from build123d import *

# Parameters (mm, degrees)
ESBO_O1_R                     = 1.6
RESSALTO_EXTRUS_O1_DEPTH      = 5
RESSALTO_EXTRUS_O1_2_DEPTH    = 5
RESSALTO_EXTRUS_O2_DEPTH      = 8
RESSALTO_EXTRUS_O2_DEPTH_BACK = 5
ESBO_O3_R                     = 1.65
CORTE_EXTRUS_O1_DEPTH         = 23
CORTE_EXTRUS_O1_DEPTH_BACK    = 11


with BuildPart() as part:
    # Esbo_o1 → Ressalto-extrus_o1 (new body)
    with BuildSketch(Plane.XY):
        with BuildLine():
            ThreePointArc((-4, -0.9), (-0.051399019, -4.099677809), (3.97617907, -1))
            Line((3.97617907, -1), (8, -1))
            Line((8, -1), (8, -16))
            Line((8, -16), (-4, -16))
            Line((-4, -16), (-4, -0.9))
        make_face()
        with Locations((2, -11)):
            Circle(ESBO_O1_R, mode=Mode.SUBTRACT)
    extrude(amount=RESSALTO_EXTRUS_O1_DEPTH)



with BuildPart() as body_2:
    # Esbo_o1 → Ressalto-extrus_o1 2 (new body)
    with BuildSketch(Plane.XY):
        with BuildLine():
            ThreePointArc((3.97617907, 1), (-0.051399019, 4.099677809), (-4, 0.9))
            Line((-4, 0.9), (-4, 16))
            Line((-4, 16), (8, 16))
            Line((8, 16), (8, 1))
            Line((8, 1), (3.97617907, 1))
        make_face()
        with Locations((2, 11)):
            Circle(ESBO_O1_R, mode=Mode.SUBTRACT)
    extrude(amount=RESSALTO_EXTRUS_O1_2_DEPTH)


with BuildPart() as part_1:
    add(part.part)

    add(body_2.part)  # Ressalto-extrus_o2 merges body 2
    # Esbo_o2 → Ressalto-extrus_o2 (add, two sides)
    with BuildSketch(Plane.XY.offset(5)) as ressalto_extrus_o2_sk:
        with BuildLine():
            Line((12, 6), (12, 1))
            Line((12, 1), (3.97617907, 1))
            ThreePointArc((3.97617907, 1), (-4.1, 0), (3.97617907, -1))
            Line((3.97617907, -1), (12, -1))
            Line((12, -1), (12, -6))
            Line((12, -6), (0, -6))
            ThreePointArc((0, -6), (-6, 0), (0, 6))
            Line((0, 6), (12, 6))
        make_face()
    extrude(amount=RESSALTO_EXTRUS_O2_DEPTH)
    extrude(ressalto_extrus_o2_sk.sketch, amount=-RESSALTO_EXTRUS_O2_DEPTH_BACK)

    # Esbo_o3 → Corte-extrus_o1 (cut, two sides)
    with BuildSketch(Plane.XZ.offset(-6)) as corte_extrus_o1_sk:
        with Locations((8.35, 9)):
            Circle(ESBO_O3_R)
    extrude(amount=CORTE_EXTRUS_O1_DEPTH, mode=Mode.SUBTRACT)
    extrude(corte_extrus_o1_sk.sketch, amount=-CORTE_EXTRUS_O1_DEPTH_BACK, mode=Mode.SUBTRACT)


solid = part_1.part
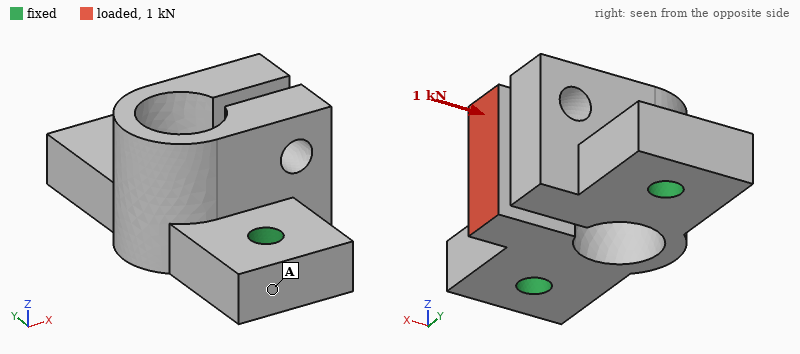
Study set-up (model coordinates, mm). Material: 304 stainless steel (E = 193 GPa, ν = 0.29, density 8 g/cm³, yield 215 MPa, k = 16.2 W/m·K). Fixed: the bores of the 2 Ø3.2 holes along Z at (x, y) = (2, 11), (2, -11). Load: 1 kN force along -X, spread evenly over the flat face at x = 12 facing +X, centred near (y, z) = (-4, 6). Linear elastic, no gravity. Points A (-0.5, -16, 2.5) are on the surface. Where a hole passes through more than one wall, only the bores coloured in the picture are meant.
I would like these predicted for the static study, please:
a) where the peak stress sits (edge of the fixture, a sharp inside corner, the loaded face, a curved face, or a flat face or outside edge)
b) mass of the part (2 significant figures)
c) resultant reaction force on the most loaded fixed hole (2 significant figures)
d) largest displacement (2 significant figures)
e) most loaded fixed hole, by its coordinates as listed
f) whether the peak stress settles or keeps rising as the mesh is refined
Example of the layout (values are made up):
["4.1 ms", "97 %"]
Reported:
["edge of the fixture", "22 g", "930 N", "18 µm", "(2, -11)", "keeps rising"]
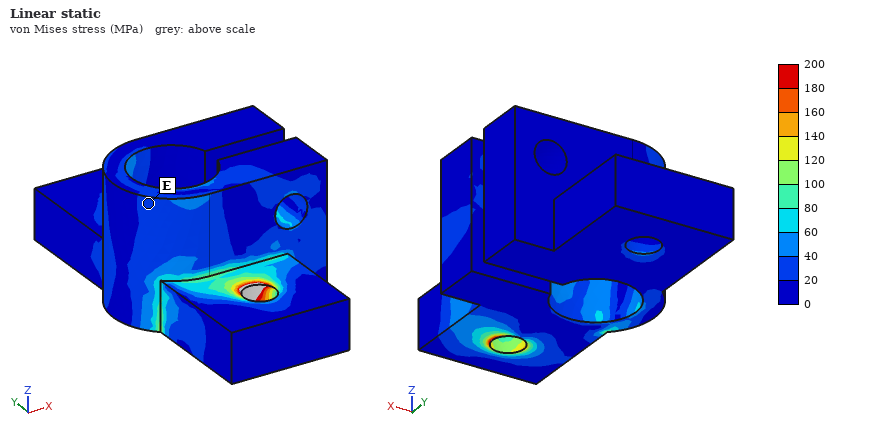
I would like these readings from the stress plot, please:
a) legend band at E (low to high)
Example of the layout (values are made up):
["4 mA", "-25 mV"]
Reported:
["20 to 40 MPa"]
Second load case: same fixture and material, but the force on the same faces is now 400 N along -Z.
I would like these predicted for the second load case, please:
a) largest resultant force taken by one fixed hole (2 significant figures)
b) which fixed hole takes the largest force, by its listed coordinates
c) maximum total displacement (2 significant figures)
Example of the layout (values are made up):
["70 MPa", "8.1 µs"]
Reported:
["420 N", "(2, -11)", "18 µm"]
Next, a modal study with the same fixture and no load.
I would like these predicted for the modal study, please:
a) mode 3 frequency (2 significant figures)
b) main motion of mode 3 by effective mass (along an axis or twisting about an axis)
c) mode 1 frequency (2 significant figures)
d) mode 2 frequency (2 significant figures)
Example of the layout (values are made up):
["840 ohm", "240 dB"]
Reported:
["17 kHz", "along X", "15 kHz", "15 kHz"]
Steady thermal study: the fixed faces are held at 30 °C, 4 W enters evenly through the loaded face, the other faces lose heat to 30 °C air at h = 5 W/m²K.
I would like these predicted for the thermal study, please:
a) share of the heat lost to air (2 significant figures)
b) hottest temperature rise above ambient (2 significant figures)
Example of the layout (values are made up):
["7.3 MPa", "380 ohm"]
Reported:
["3.4 %", "70 K"]
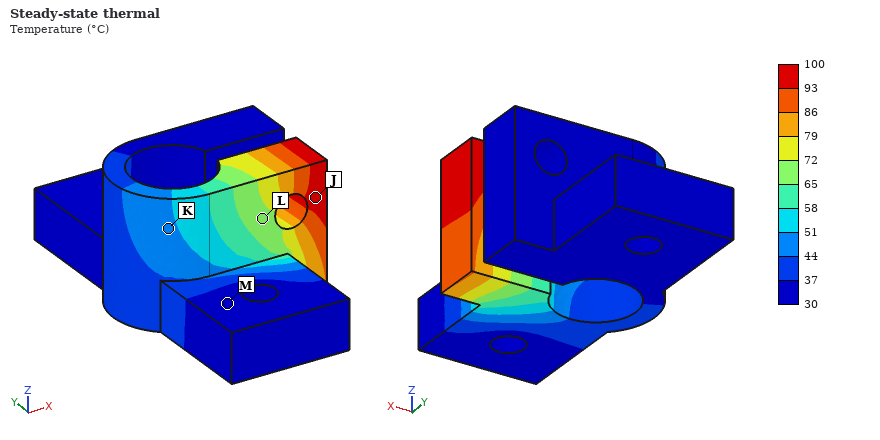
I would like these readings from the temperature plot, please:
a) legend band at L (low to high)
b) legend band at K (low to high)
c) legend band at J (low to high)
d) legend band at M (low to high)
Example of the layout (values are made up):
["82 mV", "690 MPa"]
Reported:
["65 to 72 °C", "44 to 51 °C", "93 to 100 °C", "30 to 37 °C"]
